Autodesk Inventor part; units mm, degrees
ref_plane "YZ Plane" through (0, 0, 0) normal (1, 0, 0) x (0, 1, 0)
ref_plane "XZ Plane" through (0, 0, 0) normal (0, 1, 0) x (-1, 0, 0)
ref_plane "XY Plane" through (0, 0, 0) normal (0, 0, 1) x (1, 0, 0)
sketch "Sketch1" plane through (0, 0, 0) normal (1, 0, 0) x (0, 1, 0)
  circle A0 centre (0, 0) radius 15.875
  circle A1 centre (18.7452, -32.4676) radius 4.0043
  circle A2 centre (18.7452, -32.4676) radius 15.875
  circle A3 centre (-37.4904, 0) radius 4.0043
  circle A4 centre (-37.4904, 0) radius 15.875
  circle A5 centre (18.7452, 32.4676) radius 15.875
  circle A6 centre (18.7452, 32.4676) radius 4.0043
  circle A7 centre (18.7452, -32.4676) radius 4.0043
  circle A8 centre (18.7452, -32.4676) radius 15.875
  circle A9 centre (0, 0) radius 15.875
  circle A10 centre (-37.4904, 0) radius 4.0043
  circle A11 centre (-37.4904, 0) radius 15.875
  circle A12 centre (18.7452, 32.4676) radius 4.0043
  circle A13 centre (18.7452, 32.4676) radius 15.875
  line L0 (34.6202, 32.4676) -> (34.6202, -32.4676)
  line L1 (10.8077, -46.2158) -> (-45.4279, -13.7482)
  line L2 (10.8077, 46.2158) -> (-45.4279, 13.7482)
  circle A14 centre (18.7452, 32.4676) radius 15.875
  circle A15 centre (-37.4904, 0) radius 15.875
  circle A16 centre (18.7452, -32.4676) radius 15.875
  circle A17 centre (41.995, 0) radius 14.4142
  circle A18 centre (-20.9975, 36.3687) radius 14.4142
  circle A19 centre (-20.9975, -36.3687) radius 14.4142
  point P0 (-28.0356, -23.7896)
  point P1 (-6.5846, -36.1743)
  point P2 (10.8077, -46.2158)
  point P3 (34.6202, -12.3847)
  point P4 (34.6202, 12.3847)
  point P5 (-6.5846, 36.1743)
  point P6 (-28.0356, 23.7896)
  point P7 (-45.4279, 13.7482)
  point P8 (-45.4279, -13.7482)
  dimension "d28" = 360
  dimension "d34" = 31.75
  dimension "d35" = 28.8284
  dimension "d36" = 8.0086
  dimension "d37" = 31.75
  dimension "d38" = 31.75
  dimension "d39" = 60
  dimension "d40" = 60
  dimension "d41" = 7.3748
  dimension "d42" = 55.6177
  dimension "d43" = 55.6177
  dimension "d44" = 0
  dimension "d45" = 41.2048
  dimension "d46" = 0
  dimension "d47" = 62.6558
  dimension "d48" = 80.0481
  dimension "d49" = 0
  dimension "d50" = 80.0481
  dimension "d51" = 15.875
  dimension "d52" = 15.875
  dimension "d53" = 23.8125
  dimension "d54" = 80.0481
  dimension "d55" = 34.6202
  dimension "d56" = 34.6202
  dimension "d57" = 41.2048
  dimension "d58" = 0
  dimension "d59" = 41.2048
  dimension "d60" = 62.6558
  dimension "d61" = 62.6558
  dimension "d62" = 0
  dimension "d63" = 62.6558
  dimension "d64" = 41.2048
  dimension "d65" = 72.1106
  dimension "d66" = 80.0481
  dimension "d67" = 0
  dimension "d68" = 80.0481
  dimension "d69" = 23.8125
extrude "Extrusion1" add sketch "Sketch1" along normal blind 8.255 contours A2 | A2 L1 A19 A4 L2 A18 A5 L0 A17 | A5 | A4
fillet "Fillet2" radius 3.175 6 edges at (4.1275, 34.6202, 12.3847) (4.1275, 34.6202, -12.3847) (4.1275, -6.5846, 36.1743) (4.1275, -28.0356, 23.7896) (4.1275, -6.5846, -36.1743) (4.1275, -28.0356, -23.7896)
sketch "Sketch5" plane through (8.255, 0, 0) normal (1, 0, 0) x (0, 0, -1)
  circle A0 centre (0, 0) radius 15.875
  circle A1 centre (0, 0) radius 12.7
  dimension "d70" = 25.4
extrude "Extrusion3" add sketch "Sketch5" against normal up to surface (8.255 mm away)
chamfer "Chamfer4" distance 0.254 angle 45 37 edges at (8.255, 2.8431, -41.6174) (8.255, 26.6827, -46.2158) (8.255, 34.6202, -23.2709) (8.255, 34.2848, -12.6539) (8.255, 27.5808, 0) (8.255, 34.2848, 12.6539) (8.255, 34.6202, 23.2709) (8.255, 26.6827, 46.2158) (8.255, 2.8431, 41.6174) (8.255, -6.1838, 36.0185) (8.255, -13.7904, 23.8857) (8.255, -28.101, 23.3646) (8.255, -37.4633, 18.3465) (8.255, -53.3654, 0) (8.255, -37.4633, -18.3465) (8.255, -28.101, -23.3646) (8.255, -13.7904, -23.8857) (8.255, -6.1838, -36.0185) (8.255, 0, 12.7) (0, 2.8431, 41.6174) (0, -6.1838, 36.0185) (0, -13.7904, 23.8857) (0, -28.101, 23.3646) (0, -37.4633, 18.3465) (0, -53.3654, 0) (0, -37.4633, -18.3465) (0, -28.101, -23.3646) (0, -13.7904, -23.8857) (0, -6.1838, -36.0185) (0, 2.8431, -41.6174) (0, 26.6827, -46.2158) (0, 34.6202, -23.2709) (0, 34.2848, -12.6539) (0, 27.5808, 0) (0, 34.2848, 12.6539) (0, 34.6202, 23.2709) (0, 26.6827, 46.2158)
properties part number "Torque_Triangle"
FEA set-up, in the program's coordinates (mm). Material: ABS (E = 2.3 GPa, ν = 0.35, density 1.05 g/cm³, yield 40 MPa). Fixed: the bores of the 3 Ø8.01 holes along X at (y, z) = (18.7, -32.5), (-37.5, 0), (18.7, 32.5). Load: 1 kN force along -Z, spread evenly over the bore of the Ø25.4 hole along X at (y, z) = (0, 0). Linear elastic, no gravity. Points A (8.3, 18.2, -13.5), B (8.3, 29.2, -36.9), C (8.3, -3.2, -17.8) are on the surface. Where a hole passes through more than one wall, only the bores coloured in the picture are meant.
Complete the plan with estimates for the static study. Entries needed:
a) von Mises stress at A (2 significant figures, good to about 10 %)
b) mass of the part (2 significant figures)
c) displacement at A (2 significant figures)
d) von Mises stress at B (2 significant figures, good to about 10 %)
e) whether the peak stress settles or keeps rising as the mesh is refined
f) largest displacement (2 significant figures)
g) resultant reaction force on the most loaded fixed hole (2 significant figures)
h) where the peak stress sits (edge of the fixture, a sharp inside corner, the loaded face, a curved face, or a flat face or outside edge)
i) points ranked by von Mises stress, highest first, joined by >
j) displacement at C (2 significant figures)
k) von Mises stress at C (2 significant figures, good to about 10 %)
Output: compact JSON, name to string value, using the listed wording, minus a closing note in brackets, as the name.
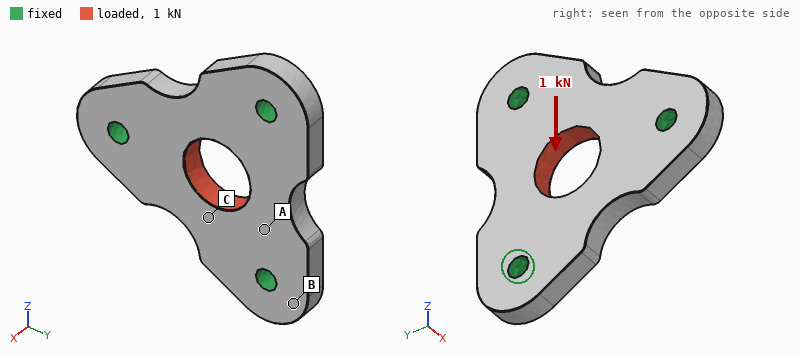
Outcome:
{"von Mises stress at A": "1.7 MPa", "mass of the part": "41 g", "displacement at A": "14 µm", "von Mises stress at B": "0.72 MPa", "whether the peak stress settles or keeps rising as the mesh is refined": "keeps rising", "largest displacement": "58 µm", "resultant reaction force on the most loaded fixed hole": "390 N", "where the peak stress sits": "edge of the fixture", "points ranked by von Mises stress, highest first, joined by >": "C > A > B", "displacement at C": "45 µm", "von Mises stress at C": "2.6 MPa"}
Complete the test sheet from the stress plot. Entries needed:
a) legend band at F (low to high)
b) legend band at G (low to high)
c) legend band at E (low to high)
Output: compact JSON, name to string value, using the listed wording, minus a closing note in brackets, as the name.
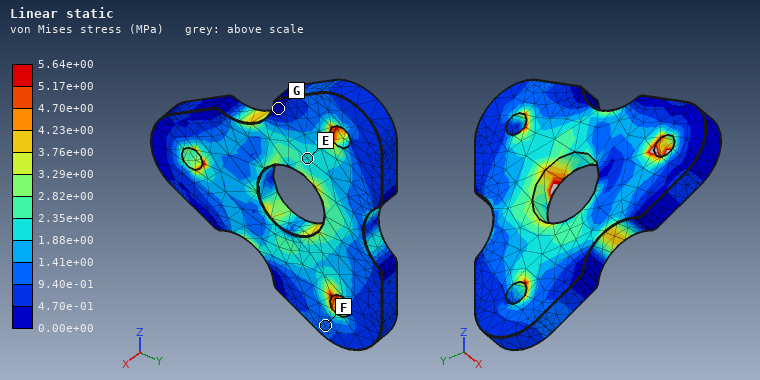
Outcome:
{"legend band at F": "9.40e-01 to 1.41e+00 MPa", "legend band at G": "0.00e+00 to 4.70e-01 MPa", "legend band at E": "1.88e+00 to 2.35e+00 MPa"}
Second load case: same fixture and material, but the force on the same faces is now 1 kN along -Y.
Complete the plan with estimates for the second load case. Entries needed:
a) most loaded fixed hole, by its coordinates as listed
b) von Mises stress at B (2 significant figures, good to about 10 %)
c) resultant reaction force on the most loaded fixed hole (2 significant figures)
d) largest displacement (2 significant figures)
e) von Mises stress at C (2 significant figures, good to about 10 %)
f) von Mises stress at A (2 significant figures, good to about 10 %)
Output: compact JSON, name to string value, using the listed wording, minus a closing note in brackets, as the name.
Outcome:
{"most loaded fixed hole, by its coordinates as listed": "(-37.5, 0)", "von Mises stress at B": "0.76 MPa", "resultant reaction force on the most loaded fixed hole": "430 N", "largest displacement": "64 µm", "von Mises stress at C": "1.4 MPa", "von Mises stress at A": "1.8 MPa"}
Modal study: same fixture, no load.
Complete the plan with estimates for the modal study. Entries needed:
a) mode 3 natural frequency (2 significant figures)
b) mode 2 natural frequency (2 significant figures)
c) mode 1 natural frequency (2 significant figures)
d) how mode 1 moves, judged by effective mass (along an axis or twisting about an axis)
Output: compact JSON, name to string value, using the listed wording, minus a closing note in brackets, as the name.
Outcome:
{"mode 3 natural frequency": "3300 Hz", "mode 2 natural frequency": "3300 Hz", "mode 1 natural frequency": "2900 Hz", "how mode 1 moves, judged by effective mass": "along X"}
